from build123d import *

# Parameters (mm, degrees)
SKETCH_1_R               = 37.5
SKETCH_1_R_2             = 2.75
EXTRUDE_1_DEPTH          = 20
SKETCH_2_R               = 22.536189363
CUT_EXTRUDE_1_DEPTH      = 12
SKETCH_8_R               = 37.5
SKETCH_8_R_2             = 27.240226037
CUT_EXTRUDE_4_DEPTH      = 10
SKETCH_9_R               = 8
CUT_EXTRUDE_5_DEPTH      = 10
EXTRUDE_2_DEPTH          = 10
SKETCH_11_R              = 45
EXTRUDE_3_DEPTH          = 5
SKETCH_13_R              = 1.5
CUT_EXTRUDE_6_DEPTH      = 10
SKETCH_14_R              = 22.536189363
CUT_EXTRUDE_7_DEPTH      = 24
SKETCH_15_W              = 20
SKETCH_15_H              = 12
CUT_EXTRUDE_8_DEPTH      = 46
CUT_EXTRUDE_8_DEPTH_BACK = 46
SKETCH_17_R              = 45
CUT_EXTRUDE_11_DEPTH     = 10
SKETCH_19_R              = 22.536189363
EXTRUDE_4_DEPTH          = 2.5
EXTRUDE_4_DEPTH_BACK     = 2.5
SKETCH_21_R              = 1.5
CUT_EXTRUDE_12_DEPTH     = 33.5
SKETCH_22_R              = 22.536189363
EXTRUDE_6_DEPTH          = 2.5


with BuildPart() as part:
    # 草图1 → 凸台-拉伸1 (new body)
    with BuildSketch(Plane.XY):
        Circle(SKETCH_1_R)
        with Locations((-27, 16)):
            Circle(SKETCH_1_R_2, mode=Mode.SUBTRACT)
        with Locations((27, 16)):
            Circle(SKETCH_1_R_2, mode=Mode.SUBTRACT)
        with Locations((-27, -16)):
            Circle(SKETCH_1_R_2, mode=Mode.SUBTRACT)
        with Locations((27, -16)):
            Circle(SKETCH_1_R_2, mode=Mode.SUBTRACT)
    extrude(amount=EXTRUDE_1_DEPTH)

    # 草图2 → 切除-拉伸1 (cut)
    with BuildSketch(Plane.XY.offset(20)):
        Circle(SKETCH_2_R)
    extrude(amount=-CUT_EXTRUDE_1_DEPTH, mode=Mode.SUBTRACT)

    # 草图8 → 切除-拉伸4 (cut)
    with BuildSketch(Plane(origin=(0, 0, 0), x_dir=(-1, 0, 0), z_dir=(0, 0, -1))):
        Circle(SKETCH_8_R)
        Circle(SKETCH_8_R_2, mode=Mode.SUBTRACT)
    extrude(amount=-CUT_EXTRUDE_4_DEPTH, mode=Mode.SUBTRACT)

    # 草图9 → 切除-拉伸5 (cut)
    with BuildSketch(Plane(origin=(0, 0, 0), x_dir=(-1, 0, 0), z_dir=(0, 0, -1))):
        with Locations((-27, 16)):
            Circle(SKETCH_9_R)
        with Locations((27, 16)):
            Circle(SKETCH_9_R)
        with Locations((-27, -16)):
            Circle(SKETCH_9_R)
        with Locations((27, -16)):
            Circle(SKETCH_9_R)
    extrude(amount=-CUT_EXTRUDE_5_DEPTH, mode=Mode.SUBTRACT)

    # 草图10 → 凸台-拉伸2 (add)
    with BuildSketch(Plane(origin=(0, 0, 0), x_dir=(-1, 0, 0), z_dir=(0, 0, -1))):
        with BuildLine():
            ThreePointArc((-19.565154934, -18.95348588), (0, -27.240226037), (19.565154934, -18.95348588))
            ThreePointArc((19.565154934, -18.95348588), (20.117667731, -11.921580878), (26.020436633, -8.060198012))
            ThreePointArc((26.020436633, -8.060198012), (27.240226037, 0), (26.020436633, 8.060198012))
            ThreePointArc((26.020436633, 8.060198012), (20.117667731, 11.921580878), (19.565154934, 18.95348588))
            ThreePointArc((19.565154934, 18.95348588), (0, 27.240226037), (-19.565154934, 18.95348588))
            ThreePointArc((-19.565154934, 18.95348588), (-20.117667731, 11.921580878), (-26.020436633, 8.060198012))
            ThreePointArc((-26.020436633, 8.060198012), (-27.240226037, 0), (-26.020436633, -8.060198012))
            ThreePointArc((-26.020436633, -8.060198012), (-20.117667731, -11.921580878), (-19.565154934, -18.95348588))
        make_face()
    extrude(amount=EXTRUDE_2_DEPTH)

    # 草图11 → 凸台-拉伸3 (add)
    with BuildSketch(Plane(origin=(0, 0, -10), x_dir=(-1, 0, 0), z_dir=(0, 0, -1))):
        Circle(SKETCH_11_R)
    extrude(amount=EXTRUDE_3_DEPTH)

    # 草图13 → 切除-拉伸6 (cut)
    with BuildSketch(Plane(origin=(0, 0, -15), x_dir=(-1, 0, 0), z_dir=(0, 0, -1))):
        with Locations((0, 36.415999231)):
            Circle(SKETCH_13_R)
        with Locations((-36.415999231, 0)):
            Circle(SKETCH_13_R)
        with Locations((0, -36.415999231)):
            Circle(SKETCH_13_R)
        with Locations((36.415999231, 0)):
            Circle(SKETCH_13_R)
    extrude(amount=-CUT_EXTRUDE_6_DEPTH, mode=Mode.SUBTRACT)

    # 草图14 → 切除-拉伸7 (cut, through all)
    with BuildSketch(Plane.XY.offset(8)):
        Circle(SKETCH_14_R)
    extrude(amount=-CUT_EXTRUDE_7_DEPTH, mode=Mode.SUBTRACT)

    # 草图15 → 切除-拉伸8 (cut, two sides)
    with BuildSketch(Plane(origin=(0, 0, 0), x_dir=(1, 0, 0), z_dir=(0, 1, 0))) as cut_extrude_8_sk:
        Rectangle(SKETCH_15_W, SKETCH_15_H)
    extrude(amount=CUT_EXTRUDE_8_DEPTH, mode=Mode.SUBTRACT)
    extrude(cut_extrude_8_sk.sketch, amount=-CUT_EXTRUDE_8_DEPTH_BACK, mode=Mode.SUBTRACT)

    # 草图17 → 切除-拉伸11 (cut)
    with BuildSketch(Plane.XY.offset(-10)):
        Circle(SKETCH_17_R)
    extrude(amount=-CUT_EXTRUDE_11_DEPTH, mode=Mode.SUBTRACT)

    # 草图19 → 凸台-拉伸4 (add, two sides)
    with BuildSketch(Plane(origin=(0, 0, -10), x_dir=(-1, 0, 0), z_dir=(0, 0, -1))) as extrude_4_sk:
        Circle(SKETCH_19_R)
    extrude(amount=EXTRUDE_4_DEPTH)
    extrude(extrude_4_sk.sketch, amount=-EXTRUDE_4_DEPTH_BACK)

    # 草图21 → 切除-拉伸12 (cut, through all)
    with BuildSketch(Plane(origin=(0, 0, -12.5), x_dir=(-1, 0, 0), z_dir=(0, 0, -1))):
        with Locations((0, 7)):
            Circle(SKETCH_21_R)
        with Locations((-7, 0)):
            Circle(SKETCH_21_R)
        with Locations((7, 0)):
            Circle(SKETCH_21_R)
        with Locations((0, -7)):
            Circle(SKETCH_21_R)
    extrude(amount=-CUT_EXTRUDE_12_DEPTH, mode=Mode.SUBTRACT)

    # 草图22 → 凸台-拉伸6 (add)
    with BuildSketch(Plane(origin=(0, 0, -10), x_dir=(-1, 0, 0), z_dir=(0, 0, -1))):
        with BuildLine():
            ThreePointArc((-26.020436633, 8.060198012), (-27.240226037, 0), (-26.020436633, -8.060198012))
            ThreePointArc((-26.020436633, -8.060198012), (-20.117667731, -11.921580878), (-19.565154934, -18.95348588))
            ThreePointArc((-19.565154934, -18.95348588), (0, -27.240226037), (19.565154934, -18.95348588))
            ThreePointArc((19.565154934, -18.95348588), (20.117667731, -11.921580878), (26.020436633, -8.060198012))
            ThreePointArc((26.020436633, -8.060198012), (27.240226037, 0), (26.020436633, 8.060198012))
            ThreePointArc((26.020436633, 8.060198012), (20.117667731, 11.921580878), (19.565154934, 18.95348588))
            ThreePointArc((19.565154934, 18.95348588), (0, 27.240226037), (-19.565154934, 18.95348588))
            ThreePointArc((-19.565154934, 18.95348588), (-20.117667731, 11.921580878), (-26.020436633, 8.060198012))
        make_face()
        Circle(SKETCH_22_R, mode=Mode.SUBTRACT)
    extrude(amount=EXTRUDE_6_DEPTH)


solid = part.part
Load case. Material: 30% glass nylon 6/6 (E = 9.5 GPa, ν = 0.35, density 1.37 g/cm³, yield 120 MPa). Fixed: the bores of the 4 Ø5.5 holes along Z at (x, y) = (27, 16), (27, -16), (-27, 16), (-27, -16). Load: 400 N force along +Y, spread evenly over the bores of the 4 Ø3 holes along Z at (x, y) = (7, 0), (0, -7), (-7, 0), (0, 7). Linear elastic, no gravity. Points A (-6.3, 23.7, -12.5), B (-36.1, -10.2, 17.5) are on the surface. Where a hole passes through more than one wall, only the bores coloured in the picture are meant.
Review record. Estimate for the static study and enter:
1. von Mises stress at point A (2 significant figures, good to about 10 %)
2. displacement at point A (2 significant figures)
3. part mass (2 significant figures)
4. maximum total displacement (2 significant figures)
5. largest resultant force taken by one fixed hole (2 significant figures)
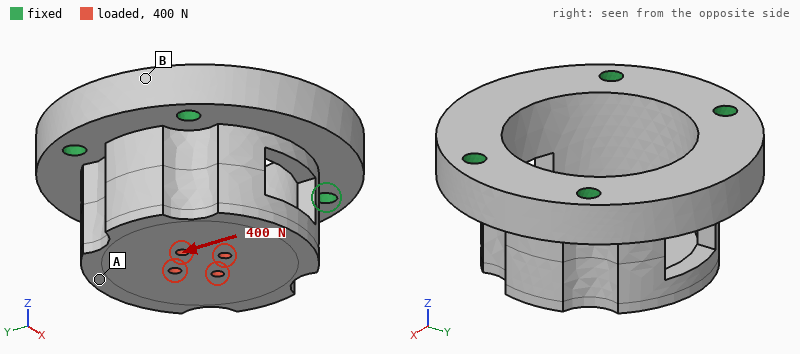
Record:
1.3 MPa
25 µm
63 g
26 µm
170 N
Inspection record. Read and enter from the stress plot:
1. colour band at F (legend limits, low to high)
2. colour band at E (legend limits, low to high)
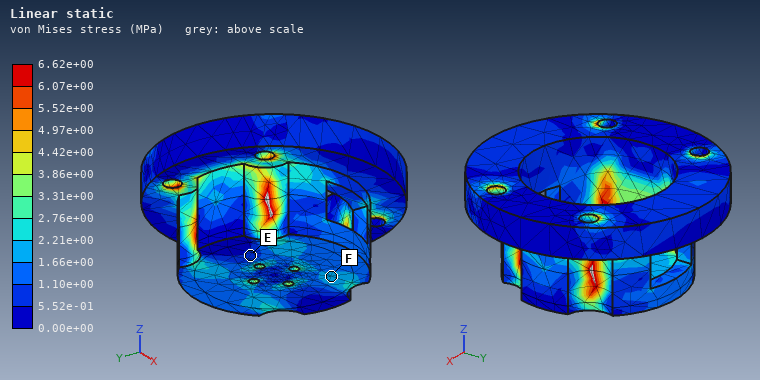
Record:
1.66e+00 to 2.21e+00 MPa
5.52e-01 to 1.10e+00 MPa
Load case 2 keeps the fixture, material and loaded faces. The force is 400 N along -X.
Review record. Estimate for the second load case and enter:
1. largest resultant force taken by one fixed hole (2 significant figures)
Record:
140 N
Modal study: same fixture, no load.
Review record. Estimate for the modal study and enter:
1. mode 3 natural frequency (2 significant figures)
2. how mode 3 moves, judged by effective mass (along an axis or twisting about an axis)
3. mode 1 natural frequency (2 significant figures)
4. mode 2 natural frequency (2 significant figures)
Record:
6000 Hz
along Z
4400 Hz
4500 Hz
